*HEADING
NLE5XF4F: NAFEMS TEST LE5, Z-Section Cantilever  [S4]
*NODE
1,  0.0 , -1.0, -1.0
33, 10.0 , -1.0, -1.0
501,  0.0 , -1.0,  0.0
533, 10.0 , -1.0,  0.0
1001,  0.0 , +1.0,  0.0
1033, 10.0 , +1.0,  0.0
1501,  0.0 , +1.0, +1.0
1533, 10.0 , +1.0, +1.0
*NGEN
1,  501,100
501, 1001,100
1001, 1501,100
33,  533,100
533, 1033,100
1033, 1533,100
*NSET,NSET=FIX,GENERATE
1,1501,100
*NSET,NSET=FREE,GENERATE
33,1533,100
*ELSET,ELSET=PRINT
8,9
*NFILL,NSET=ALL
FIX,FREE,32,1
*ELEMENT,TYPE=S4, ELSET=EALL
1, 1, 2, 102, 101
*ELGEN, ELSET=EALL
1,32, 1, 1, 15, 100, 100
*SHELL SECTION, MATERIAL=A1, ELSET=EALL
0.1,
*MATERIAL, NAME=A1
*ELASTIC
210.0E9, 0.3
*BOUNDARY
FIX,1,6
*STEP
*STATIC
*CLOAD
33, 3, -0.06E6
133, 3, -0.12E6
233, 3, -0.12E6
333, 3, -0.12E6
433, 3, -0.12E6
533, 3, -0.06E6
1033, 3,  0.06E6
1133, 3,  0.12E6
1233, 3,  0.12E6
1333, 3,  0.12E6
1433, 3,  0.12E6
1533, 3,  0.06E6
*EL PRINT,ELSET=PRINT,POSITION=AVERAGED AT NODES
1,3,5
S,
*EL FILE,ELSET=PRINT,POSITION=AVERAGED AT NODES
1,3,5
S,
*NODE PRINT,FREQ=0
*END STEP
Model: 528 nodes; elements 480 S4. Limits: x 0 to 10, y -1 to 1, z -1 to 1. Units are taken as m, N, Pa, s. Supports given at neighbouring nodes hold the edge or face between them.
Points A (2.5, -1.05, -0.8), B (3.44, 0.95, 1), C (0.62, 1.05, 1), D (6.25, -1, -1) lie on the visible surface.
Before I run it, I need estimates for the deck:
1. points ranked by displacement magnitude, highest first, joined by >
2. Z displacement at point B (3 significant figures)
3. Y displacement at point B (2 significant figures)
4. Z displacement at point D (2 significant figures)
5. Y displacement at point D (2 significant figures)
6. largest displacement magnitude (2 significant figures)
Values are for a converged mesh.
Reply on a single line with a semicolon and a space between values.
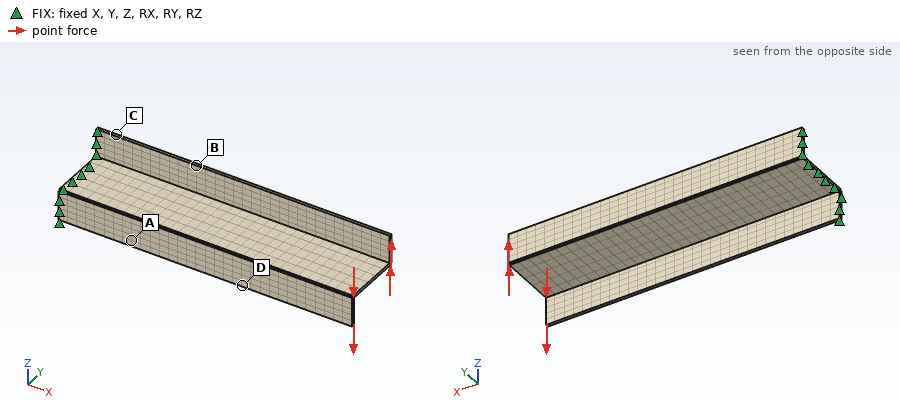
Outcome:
D > B > A > C; 0.00515 m; -0.0058 m; -0.015 m; 0.016 m; 0.044 m
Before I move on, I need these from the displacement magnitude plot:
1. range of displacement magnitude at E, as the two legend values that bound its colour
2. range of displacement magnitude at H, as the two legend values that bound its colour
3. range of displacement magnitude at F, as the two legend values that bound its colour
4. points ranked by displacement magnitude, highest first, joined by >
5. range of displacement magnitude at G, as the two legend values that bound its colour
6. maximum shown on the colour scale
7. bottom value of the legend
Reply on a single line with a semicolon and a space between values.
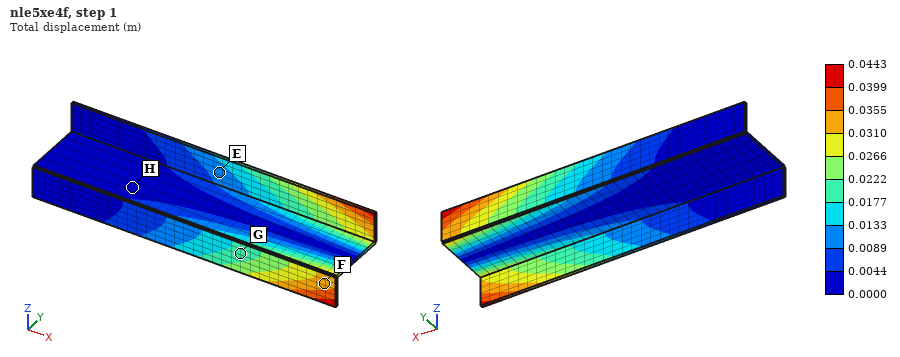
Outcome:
0.0089 to 0.0133 m; 0.0000 to 0.0044 m; 0.0310 to 0.0355 m; F > G > E > H; 0.0177 to 0.0222 m; 0.0443 m; 0.0000 m
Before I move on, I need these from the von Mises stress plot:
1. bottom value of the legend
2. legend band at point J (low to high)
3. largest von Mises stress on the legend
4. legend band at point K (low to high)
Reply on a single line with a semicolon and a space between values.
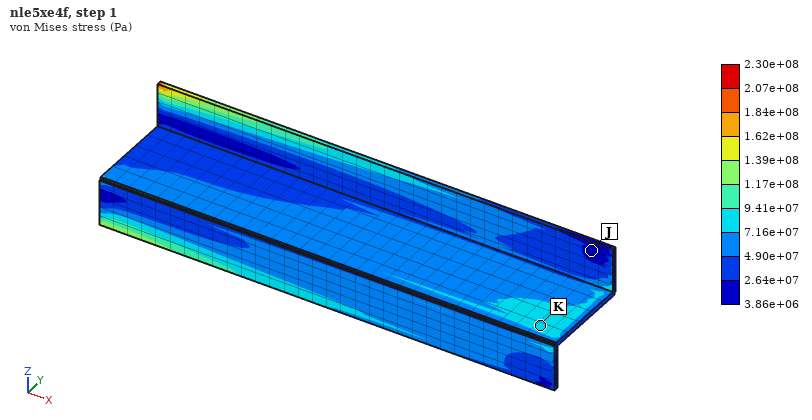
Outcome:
3.86e+06 Pa; 3.86e+06 to 2.64e+07 Pa; 2.30e+08 Pa; 7.16e+07 to 9.41e+07 Pa
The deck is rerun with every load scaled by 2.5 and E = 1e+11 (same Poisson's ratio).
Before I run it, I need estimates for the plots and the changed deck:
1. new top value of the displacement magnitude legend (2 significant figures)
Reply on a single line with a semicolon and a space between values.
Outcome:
0.23 m
